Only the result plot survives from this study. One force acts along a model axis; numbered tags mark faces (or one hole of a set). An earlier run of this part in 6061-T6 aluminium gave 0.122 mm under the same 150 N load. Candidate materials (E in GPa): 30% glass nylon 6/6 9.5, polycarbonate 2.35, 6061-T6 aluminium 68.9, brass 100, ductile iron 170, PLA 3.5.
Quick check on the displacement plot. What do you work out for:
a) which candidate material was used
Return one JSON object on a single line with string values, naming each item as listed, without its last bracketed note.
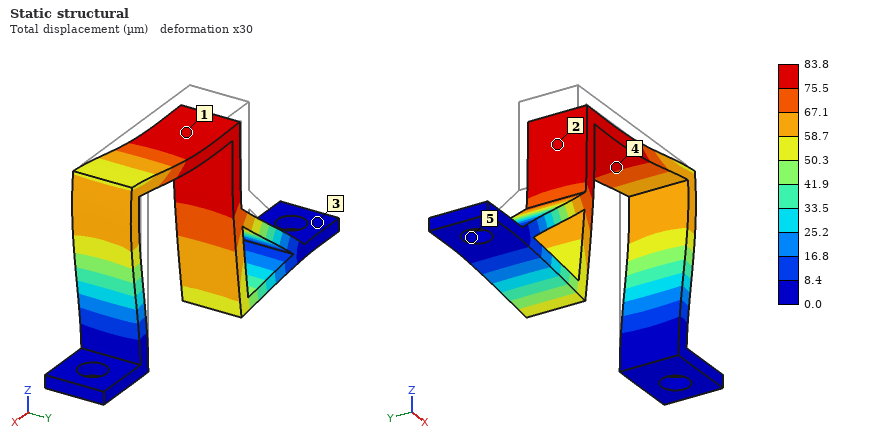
{"which candidate material was used": "brass"}
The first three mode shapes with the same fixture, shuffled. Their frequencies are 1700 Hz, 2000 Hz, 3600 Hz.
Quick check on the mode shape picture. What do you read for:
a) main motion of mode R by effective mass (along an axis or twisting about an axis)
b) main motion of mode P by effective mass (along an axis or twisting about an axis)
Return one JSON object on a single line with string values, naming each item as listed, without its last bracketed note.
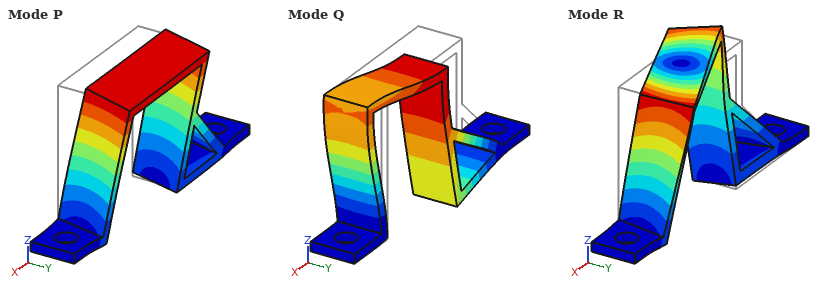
{"main motion of mode R by effective mass": "twisting about Z", "main motion of mode P by effective mass": "along Y"}
